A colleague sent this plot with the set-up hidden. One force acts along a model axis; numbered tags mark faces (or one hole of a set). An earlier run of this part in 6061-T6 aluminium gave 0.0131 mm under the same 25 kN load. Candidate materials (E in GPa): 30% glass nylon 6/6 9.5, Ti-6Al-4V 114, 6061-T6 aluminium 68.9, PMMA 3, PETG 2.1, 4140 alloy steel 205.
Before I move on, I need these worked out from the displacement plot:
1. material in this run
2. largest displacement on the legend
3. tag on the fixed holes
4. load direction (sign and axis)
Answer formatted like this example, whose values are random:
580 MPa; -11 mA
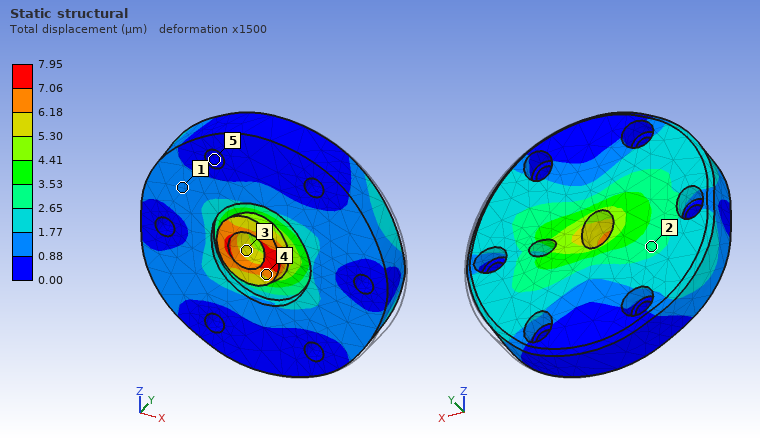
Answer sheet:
Ti-6Al-4V; 7.95 µm; 5; -X
